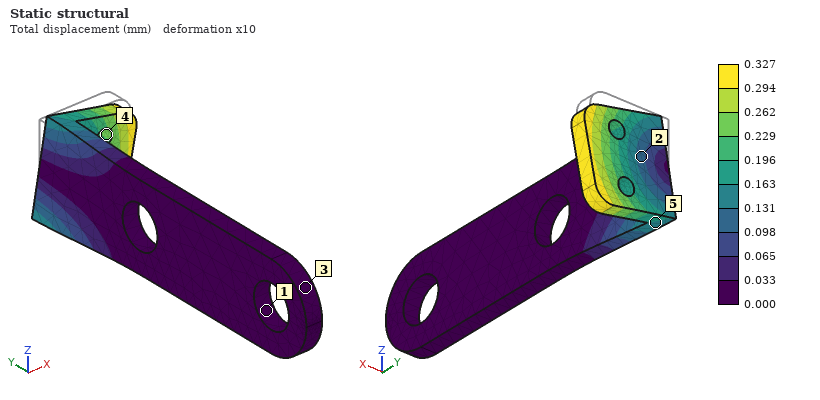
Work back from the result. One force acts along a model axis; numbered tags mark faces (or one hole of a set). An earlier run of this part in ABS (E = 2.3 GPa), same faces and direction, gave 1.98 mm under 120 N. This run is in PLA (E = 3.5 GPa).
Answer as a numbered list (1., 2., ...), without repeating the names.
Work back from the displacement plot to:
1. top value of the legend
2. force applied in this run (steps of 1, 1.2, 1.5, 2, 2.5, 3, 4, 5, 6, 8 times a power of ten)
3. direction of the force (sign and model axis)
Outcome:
1. 0.327 mm
2. 30 N
3. -Z
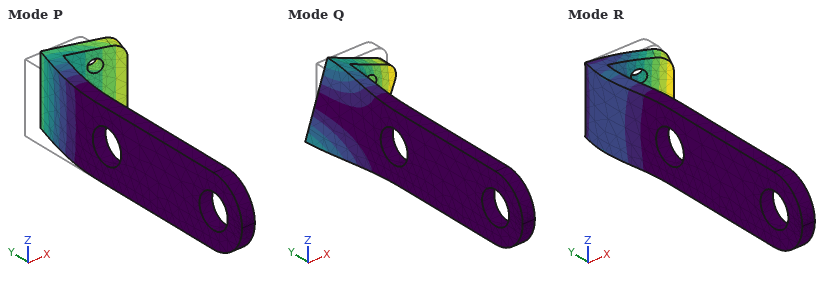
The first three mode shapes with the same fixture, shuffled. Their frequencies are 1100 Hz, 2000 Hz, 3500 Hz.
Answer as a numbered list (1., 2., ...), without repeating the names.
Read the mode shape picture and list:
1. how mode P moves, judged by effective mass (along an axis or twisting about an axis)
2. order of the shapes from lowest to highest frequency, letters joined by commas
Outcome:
1. along X
2. P, Q, R
